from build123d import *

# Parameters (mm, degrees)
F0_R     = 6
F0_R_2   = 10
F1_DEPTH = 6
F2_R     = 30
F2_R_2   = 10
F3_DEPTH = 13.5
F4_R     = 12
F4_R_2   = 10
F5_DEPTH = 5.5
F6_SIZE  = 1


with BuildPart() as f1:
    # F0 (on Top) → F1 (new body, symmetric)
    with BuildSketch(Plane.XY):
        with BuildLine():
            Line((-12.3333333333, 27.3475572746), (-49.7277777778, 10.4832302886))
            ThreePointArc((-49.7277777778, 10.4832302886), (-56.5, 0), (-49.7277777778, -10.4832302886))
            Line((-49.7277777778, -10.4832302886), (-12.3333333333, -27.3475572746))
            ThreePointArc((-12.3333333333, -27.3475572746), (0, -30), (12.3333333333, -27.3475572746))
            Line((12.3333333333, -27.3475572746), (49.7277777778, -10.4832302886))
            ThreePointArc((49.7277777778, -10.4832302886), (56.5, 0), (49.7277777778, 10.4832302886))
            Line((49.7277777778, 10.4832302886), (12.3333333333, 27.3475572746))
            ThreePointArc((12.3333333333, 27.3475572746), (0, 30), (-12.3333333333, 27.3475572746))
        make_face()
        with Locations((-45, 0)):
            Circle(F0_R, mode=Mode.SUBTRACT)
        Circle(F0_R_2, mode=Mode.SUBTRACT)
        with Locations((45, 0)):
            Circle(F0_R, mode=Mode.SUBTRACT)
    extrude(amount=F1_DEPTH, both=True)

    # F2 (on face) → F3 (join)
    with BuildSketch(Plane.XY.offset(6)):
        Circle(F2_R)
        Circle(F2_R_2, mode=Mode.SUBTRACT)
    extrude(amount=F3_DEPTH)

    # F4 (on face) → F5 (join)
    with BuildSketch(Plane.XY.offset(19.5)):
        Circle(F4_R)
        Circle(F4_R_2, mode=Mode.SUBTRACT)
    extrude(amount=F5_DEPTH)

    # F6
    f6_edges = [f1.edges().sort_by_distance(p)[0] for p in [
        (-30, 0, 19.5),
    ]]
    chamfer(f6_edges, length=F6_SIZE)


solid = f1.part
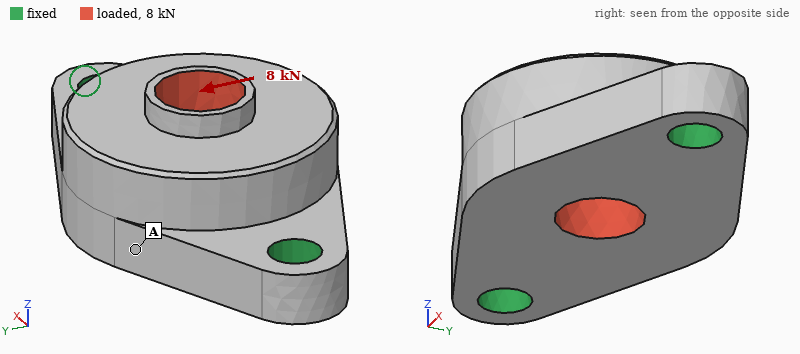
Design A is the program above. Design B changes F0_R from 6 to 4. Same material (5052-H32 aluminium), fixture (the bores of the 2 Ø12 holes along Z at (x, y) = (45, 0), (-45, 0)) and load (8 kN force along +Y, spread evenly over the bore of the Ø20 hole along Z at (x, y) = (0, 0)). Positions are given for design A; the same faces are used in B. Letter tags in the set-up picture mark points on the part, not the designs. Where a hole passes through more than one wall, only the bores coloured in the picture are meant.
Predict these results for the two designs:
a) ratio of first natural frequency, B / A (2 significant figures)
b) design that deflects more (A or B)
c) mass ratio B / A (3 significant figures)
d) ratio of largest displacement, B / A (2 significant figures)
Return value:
0.88
B
1.02
1.3
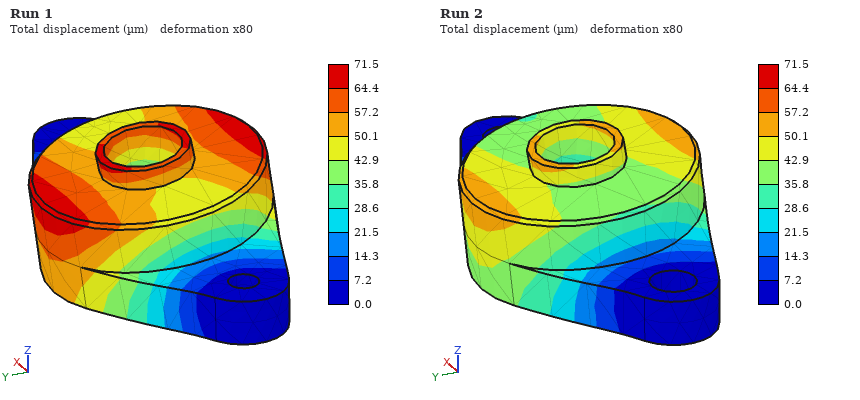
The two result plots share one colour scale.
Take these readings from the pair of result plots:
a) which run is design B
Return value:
Run 1
